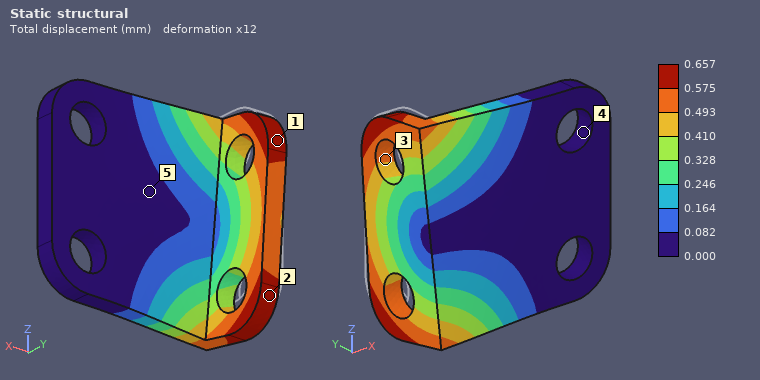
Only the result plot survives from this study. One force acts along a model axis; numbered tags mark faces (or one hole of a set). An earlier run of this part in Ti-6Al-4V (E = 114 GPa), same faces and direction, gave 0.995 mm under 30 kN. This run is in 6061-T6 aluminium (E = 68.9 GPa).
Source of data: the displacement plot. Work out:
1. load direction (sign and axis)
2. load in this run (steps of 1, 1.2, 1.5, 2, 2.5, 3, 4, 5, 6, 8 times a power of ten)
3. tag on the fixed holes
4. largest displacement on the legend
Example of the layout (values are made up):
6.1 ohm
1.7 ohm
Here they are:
-Z
12 kN
4
0.657 mm
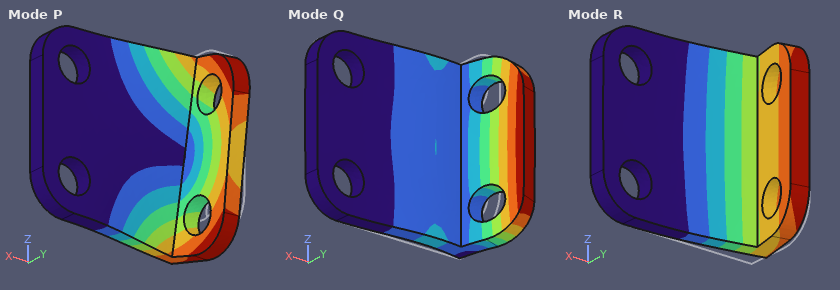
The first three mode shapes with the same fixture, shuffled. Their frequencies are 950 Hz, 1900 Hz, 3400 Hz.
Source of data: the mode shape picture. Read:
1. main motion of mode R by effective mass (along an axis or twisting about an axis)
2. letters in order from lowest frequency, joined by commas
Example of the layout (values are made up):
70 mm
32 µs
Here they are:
along Y
R, P, Q
